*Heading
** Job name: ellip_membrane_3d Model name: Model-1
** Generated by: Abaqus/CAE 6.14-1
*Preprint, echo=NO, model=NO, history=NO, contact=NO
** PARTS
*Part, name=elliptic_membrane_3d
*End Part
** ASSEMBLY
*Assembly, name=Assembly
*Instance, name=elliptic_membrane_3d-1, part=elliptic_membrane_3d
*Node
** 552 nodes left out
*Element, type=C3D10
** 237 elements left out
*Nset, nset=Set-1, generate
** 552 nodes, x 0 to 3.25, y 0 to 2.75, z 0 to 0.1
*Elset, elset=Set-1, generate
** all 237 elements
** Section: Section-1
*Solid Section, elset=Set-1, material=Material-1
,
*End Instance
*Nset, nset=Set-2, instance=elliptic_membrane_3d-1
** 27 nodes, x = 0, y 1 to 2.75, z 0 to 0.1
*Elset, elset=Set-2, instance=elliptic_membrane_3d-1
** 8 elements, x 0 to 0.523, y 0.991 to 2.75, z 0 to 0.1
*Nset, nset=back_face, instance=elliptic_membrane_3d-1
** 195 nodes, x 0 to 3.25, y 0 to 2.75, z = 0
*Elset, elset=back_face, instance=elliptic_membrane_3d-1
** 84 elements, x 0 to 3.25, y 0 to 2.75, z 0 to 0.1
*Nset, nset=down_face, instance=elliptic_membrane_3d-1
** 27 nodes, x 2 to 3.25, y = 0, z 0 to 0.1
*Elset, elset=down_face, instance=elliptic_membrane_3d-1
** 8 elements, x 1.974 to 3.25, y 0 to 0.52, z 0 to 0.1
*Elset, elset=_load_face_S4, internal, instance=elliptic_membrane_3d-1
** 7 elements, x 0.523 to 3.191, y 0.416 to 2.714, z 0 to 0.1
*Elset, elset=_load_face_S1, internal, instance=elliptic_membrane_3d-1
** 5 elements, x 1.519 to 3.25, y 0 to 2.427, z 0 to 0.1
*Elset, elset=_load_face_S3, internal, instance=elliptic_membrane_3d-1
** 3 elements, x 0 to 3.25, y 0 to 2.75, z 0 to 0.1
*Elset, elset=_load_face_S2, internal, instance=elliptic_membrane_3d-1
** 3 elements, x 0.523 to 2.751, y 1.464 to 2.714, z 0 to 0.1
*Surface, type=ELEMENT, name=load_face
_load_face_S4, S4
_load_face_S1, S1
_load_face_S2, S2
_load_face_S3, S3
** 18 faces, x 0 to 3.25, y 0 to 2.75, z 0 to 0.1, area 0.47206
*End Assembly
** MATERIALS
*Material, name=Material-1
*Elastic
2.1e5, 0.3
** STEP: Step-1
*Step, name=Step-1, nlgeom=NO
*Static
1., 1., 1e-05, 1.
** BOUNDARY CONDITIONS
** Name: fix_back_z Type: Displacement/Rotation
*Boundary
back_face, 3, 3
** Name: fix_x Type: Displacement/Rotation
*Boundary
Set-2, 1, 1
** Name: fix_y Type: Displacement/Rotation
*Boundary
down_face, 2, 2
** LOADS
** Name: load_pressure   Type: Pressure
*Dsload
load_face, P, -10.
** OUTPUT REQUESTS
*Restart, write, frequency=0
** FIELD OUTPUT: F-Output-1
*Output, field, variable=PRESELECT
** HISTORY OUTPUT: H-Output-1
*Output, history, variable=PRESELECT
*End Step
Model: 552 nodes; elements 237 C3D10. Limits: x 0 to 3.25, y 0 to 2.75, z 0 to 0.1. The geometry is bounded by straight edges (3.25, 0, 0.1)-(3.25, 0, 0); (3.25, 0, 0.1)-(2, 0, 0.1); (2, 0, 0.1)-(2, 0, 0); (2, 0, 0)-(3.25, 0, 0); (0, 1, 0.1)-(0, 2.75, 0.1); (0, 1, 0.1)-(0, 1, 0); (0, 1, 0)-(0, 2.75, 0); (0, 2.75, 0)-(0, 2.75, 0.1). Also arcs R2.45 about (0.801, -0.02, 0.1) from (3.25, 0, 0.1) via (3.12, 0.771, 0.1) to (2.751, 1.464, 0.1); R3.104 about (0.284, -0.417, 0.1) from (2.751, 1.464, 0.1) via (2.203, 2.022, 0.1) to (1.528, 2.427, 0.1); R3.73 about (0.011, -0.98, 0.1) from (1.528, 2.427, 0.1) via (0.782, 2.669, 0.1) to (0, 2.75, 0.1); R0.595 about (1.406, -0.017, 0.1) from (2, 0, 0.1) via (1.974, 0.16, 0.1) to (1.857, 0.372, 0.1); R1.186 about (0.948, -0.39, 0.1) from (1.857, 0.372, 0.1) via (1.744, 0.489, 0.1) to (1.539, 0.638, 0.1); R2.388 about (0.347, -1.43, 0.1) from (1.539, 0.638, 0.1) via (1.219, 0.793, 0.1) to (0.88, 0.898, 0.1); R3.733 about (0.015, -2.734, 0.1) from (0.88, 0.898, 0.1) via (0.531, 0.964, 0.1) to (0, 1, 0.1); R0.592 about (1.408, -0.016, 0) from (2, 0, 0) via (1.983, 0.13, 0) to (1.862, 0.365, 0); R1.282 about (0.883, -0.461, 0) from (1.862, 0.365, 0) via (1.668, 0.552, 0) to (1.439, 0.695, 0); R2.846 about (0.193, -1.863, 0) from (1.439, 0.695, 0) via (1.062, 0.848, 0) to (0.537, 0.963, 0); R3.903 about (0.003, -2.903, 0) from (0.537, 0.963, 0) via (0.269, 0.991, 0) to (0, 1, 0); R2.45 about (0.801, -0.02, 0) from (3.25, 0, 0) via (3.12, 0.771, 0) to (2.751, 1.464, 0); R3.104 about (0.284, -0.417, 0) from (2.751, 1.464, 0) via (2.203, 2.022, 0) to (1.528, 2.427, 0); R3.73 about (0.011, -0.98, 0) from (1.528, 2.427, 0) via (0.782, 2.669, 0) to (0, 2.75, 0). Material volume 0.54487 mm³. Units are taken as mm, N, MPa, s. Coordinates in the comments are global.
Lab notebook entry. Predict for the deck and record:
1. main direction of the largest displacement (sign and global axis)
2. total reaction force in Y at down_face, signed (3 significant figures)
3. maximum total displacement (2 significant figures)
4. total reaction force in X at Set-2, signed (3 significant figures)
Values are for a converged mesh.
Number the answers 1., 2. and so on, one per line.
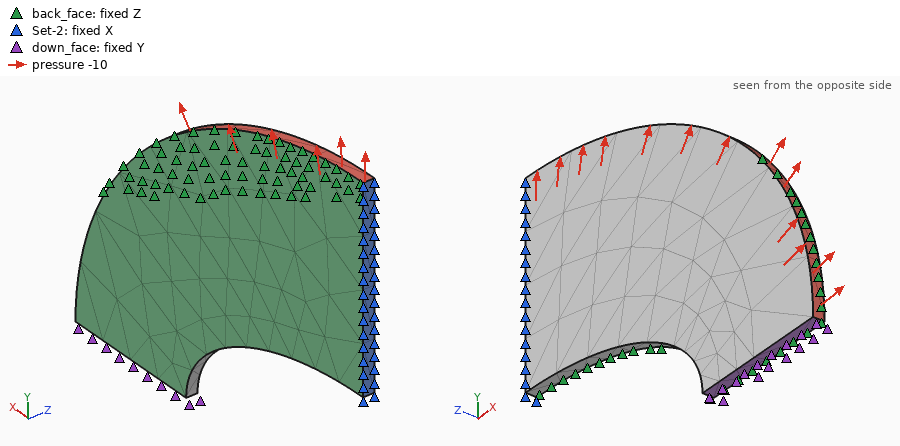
1. +Y
2. -3.25 N
3. 5.5e-04 mm
4. -2.75 N
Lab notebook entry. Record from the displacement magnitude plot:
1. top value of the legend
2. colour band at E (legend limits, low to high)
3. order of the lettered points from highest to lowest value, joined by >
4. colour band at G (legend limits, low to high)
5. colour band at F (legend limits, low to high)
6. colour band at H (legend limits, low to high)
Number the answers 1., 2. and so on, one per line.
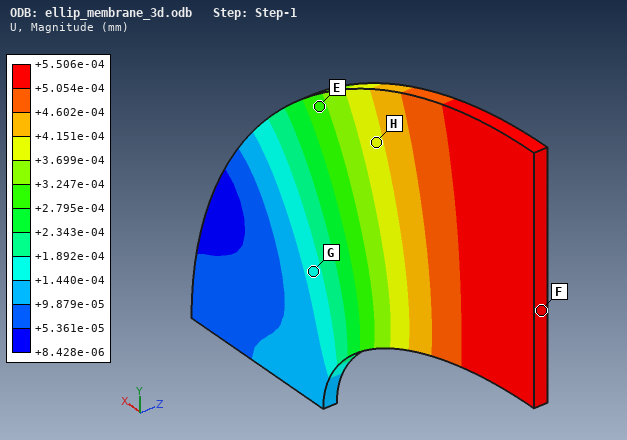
1. +5.506e-04 mm
2. +2.795e-04 to +3.247e-04 mm
3. F > H > E > G
4. +1.440e-04 to +1.892e-04 mm
5. +5.054e-04 to +5.506e-04 mm
6. +3.699e-04 to +4.151e-04 mm
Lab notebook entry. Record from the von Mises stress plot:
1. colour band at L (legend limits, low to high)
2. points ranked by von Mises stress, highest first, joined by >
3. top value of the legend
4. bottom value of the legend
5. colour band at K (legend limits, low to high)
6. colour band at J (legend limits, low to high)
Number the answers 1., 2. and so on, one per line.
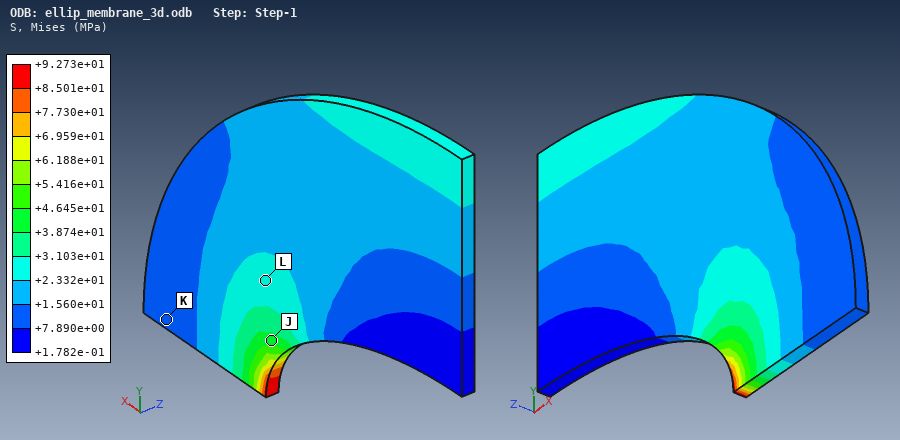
1. +2.332e+01 to +3.103e+01 MPa
2. J > L > K
3. +9.273e+01 MPa
4. +1.782e-01 MPa
5. +7.890e+00 to +1.560e+01 MPa
6. +3.874e+01 to +4.645e+01 MPa
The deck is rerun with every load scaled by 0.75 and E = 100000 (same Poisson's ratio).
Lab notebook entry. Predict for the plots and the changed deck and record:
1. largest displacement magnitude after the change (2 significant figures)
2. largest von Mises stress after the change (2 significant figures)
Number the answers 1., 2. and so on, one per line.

1. 8.7e-04 mm
2. 70 MPa
